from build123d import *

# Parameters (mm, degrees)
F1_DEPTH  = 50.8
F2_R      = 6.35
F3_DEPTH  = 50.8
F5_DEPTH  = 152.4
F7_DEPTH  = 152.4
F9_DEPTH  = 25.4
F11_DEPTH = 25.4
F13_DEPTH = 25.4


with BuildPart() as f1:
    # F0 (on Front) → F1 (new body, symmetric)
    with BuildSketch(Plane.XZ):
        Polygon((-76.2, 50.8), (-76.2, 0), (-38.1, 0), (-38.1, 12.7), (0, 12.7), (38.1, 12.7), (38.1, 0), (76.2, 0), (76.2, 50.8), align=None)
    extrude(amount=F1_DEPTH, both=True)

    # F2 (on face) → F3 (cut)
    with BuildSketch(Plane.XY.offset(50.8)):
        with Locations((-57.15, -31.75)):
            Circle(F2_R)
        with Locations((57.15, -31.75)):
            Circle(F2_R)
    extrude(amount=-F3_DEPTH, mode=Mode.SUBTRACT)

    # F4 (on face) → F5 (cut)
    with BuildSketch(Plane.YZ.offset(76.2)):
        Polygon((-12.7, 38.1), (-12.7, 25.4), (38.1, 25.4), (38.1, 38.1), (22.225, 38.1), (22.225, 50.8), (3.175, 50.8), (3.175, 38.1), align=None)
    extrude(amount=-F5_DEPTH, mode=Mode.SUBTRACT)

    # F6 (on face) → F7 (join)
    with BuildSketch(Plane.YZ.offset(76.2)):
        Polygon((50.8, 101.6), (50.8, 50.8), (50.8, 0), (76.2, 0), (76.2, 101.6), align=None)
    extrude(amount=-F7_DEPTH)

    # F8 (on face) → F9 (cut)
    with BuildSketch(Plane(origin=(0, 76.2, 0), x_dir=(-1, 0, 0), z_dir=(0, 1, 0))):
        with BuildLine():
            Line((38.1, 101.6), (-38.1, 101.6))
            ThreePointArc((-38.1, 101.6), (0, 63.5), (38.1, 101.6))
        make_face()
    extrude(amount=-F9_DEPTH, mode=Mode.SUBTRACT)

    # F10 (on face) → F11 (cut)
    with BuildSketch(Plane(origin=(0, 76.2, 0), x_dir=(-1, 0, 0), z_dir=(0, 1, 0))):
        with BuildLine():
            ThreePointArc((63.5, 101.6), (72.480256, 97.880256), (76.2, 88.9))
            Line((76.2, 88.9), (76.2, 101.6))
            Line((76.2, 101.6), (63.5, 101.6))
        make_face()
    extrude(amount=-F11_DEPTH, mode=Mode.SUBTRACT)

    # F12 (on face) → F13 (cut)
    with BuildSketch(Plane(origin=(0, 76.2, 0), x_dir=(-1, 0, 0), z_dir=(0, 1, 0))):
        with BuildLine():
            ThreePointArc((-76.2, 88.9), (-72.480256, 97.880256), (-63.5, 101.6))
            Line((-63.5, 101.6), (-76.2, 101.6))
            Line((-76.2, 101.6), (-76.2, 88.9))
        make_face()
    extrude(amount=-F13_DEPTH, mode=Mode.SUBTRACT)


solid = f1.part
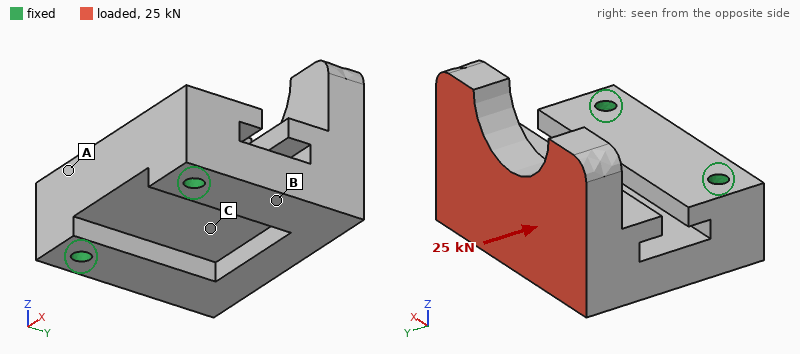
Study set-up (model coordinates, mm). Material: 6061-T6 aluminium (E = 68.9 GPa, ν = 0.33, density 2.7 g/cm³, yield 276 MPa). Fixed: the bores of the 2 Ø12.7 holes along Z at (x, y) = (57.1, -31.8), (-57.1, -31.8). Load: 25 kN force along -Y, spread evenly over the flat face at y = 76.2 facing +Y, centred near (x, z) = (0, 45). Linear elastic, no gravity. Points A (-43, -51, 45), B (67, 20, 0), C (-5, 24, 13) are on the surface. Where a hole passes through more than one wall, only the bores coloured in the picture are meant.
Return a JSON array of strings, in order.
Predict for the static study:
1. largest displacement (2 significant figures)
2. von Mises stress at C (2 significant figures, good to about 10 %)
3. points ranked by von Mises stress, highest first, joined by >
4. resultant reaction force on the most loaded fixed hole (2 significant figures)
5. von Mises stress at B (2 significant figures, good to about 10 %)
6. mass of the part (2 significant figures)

["0.66 mm", "29 MPa", "B > C > A", "14 kN", "66 MPa", "2.4 kg"]
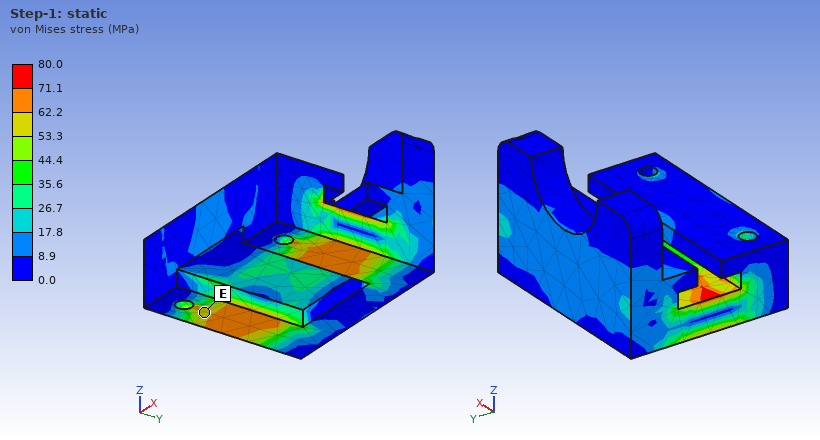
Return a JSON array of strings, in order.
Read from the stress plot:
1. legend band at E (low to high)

["53.3 to 62.2 MPa"]
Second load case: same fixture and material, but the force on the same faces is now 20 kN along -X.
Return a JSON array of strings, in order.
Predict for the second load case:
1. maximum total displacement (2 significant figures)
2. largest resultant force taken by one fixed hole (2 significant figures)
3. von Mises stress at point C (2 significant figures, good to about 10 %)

["0.14 mm", "21 kN", "14 MPa"]
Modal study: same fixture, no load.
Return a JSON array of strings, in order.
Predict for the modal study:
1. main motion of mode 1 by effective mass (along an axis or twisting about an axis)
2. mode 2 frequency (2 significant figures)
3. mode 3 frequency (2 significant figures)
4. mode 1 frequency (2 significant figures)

["along Z", "1700 Hz", "2900 Hz", "820 Hz"]
